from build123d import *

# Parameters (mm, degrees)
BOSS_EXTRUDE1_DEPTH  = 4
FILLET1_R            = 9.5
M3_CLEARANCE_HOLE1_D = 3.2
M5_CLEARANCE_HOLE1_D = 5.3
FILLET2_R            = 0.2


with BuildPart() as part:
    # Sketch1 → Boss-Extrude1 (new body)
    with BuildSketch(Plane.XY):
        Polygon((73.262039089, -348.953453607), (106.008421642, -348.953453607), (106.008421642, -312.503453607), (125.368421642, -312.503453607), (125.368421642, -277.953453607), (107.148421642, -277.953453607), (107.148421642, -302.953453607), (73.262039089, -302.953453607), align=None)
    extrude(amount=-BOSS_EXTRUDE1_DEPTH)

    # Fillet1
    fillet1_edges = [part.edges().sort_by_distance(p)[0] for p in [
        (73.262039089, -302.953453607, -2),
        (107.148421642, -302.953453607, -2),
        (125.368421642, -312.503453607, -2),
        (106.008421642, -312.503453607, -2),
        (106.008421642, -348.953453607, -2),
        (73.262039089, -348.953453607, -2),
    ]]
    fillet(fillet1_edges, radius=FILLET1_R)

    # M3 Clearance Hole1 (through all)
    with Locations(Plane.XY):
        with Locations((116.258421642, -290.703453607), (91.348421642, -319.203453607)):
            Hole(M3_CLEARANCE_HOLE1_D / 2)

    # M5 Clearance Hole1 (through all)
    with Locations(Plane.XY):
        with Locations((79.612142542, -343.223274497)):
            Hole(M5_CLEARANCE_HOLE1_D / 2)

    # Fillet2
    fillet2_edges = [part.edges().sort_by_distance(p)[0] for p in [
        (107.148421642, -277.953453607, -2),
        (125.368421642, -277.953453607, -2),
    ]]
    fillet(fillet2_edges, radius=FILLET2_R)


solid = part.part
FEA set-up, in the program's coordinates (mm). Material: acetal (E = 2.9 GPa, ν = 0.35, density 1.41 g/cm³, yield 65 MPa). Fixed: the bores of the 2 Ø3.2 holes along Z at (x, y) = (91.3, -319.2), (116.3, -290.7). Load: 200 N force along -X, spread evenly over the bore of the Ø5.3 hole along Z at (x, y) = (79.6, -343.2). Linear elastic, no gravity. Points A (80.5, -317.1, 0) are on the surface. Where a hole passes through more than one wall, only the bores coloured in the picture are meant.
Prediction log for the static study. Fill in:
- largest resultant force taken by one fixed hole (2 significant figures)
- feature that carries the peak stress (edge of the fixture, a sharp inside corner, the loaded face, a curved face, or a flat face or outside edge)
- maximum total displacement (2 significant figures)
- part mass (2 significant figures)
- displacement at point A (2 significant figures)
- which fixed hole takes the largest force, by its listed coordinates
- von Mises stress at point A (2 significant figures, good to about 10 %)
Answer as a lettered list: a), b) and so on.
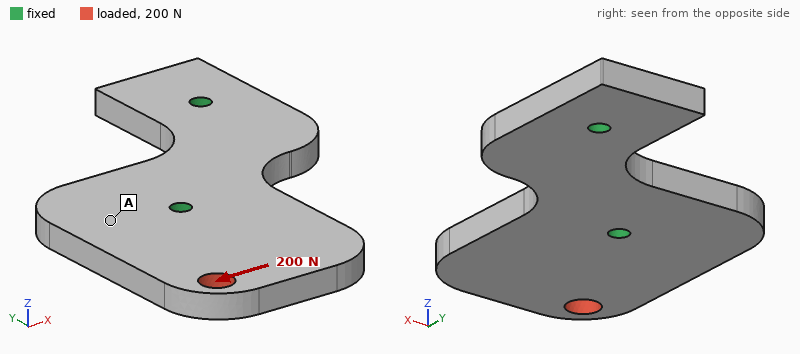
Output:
a) 260 N
b) edge of the fixture
c) 0.29 mm
d) 12 g
e) 0.080 mm
f) (91.3, -319.2)
g) 3.3 MPa
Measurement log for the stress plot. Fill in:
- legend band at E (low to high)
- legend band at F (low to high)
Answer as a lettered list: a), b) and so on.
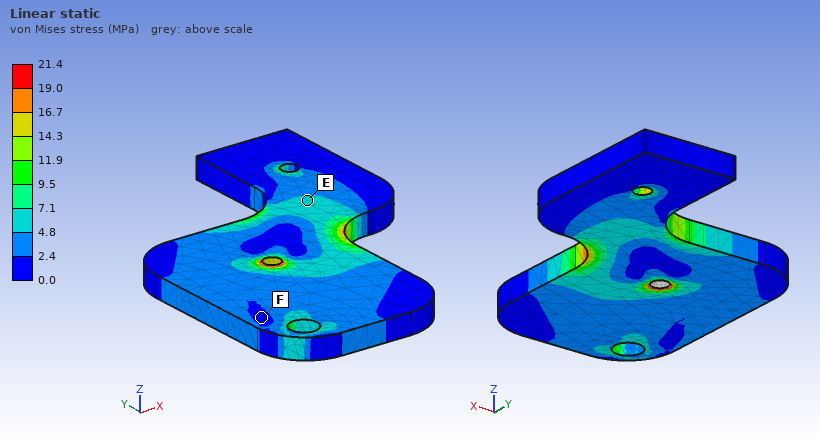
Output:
a) 4.8 to 7.1 MPa
b) 0.0 to 2.4 MPa
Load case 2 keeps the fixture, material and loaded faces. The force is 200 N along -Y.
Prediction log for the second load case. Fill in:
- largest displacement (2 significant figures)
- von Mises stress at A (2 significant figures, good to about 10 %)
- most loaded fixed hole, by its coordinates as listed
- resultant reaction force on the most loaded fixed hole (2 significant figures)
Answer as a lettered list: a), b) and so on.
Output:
a) 0.16 mm
b) 2.5 MPa
c) (91.3, -319.2)
d) 260 N
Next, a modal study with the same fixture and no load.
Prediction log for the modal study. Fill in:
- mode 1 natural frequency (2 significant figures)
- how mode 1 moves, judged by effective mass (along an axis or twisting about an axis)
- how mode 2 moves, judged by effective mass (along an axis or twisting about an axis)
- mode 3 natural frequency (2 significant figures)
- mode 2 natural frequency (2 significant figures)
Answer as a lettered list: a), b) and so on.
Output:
a) 990 Hz
b) along Z
c) twisting about Y
d) 2600 Hz
e) 1700 Hz
